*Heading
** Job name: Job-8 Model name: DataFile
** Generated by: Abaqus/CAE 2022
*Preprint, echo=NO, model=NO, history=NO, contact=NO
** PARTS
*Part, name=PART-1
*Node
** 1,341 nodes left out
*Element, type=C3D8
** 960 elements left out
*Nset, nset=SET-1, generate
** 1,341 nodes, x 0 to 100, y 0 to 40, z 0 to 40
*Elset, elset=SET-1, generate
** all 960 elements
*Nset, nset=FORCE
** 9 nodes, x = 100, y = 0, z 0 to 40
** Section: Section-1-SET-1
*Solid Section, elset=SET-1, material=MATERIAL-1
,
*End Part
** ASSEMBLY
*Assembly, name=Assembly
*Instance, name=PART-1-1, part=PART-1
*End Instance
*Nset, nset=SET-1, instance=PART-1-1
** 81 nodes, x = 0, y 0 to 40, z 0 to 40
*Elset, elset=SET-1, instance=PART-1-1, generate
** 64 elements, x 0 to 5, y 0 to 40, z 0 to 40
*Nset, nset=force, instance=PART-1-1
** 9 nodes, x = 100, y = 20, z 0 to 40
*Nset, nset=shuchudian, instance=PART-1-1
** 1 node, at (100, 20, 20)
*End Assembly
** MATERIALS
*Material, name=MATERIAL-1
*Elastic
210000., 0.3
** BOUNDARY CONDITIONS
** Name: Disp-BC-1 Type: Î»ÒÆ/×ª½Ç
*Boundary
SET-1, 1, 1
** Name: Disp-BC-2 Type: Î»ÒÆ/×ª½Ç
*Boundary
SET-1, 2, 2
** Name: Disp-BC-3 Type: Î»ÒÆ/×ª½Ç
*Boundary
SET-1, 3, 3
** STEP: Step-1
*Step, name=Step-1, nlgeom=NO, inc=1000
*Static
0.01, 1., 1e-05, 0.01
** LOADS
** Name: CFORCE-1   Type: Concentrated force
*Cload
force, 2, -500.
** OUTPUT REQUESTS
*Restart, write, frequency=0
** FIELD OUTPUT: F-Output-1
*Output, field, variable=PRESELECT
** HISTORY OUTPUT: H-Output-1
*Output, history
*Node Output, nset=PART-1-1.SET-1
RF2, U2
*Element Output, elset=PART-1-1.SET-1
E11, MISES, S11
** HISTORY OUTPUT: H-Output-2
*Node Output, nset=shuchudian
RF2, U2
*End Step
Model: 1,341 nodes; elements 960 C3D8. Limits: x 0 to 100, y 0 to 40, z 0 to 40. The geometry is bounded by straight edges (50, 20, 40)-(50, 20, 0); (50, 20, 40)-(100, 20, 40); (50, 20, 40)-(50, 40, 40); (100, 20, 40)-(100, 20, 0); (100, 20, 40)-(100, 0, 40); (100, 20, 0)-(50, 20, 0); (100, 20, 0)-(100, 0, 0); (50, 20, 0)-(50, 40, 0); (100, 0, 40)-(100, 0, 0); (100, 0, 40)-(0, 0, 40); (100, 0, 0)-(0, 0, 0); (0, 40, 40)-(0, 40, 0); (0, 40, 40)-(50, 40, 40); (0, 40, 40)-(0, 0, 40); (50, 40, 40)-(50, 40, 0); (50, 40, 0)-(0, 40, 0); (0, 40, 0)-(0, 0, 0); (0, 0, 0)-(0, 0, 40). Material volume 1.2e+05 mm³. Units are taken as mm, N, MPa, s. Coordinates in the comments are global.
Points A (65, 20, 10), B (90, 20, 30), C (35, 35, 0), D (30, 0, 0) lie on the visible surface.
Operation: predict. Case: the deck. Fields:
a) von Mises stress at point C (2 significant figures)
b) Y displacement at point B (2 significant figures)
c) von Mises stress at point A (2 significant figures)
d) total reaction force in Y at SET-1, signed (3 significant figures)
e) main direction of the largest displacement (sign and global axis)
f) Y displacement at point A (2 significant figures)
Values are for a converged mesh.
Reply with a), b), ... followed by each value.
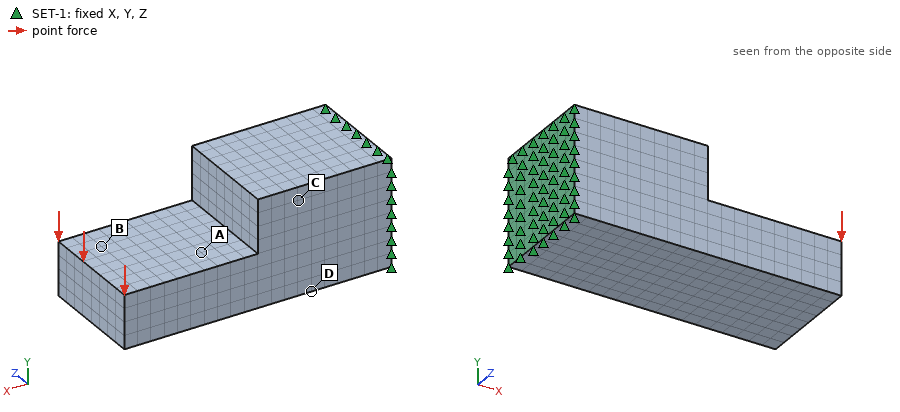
a) 20 MPa
b) -0.068 mm
c) 58 MPa
d) 4500 N
e) -Y
f) -0.029 mm
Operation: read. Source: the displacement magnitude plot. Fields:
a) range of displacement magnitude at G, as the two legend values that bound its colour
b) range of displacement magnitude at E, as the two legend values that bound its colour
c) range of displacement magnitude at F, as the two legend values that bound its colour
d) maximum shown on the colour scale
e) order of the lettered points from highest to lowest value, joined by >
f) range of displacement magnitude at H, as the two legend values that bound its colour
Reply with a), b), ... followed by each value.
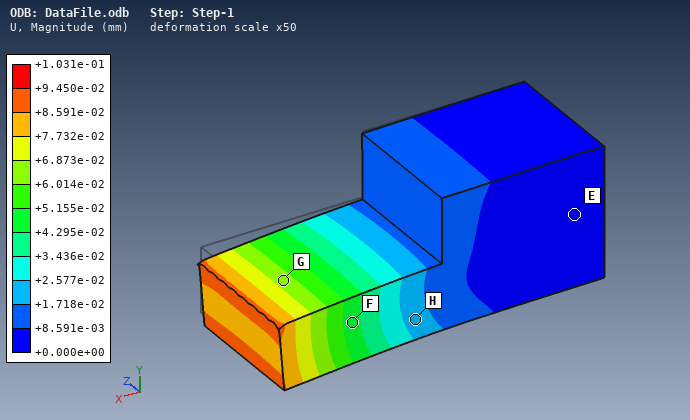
a) +6.014e-02 to +6.873e-02 mm
b) +0.000e+00 to +8.591e-03 mm
c) +4.295e-02 to +5.155e-02 mm
d) +1.031e-01 mm
e) G > F > H > E
f) +1.718e-02 to +2.577e-02 mm
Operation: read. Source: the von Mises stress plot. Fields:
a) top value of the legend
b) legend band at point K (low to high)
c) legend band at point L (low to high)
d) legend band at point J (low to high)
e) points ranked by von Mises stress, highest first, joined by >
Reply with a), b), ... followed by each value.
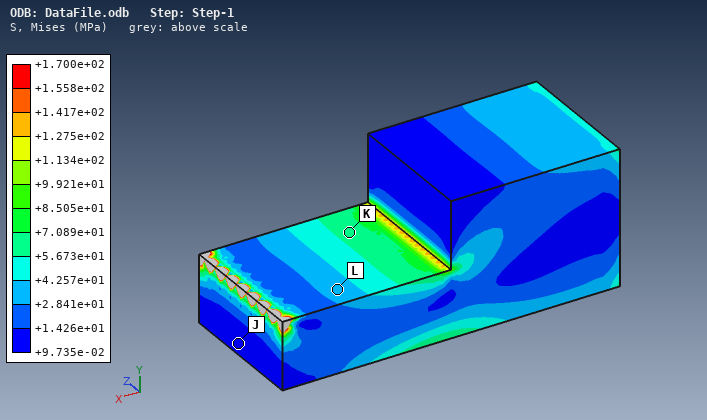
a) +1.700e+02 MPa
b) +5.673e+01 to +7.089e+01 MPa
c) +2.841e+01 to +4.257e+01 MPa
d) +9.735e-02 to +1.426e+01 MPa
e) K > L > J
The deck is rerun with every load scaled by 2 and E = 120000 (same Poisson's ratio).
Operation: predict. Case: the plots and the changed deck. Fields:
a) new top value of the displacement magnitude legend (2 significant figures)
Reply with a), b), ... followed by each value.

a) 0.36 mm
